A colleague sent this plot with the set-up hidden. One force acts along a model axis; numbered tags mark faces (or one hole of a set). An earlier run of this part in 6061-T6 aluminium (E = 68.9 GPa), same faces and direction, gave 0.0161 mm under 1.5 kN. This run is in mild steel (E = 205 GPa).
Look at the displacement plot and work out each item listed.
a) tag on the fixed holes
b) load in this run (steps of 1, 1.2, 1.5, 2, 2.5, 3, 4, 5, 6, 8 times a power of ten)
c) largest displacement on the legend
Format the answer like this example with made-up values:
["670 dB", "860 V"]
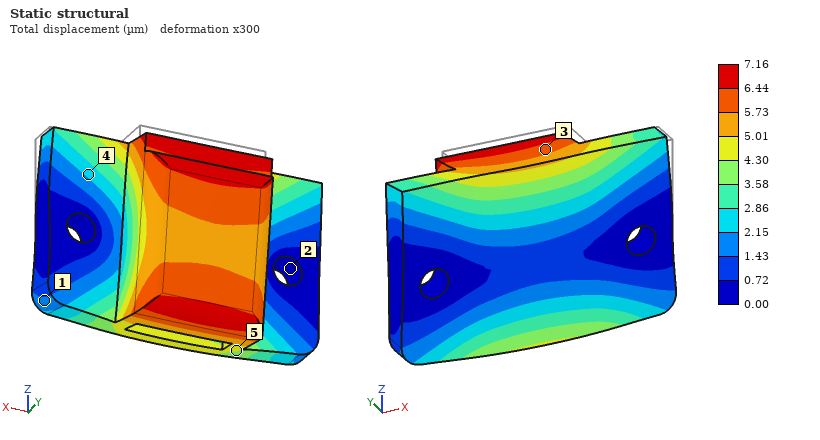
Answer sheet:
["2", "2 kN", "7.16 µm"]
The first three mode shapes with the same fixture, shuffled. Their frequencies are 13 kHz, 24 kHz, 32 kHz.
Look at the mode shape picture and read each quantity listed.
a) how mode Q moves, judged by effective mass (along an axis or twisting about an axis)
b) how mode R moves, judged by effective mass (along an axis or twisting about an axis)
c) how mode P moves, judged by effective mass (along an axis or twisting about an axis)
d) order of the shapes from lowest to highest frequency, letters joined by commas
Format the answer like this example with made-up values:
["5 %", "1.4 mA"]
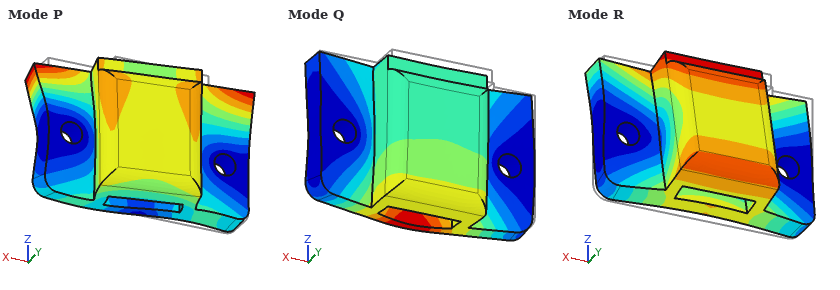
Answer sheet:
["along Y", "along Z", "along X", "R, Q, P"]
